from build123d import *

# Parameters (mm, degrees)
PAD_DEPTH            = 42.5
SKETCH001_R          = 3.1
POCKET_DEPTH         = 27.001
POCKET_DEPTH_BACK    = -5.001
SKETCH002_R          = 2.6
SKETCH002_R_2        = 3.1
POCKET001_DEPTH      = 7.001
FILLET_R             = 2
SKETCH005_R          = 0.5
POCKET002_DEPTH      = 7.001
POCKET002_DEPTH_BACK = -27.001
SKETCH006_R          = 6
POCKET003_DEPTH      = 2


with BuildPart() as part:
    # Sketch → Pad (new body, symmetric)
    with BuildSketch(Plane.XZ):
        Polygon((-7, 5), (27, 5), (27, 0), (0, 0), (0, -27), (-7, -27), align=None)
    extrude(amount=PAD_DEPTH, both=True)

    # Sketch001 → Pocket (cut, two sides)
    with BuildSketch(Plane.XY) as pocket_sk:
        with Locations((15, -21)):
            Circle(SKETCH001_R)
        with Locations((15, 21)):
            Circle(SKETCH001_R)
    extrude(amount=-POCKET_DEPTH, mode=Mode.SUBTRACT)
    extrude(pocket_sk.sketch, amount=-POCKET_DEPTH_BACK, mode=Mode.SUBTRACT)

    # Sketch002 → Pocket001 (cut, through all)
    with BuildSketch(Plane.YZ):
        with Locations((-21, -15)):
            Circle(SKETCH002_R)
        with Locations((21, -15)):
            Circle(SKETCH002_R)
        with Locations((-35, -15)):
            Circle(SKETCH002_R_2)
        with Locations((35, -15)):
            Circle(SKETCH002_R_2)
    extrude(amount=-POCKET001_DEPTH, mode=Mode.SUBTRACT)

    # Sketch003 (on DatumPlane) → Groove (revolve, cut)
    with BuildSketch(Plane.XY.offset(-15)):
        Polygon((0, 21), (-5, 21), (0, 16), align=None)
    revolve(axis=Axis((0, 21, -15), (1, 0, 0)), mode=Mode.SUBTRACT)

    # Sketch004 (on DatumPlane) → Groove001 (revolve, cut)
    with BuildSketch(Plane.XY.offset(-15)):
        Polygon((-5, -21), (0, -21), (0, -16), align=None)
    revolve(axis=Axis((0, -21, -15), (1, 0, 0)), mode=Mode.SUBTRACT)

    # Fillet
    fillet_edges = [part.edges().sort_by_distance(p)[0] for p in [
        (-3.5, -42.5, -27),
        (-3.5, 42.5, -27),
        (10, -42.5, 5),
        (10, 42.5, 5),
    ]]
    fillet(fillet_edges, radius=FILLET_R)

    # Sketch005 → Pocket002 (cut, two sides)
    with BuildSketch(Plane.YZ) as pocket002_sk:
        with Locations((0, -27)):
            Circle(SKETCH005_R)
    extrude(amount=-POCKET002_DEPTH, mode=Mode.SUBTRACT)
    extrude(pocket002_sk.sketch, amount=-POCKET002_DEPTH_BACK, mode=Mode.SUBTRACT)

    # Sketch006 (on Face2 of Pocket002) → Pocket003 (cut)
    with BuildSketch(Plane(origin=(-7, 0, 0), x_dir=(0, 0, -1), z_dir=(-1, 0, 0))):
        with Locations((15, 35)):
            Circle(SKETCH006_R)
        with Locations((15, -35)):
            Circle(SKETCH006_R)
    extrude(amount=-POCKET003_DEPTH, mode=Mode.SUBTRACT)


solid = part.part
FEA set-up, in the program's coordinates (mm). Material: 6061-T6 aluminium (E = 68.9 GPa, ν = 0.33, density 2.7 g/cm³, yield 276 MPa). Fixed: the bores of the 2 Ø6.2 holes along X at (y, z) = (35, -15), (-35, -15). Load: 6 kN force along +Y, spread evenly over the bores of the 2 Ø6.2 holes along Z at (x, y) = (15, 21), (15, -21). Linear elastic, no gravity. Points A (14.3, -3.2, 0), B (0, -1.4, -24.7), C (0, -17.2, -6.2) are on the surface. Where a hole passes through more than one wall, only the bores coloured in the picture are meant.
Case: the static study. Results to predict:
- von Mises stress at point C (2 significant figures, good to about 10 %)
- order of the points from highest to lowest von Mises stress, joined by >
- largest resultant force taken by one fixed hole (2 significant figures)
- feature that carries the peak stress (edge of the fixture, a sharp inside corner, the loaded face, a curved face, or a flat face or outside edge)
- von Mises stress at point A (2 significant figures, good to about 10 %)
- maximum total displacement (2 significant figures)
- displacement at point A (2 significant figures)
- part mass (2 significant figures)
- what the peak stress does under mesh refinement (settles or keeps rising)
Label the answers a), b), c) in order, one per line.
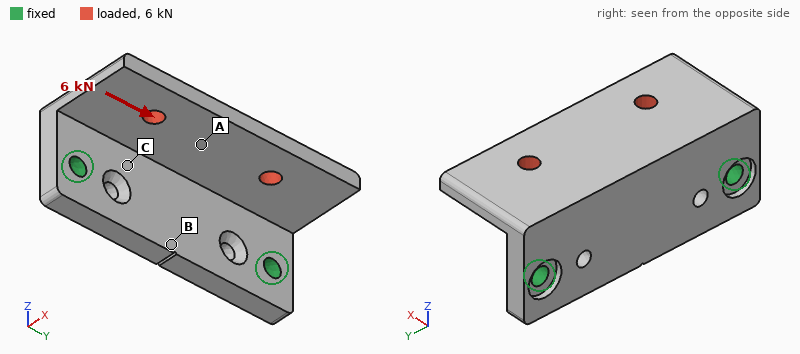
a) 62 MPa
b) C > A > B
c) 3.6 kN
d) edge of the fixture
e) 37 MPa
f) 0.16 mm
g) 0.060 mm
h) 78 g
i) keeps rising
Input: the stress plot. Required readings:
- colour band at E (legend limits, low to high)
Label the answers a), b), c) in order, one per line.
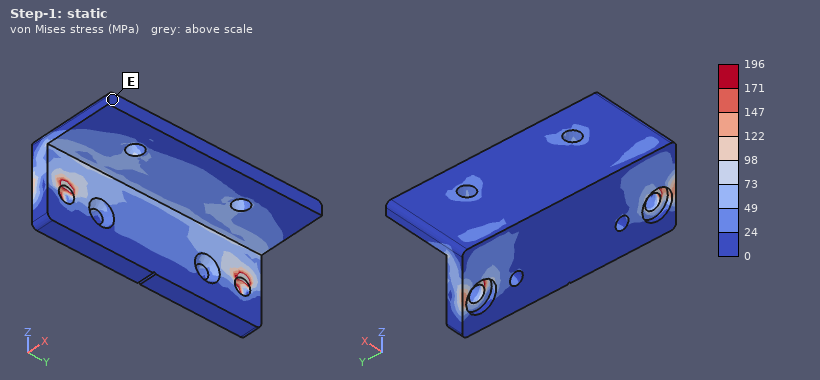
a) 0 to 24 MPa
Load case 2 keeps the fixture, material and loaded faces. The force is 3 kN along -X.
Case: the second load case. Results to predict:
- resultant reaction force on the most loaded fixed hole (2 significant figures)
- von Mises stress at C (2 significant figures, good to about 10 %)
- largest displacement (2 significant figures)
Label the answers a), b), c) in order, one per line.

a) 1.5 kN
b) 21 MPa
c) 0.22 mm
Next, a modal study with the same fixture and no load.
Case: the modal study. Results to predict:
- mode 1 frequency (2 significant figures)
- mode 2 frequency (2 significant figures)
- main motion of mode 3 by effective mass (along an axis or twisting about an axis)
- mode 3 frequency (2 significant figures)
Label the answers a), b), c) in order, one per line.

a) 2600 Hz
b) 4400 Hz
c) along X
d) 5900 Hz
